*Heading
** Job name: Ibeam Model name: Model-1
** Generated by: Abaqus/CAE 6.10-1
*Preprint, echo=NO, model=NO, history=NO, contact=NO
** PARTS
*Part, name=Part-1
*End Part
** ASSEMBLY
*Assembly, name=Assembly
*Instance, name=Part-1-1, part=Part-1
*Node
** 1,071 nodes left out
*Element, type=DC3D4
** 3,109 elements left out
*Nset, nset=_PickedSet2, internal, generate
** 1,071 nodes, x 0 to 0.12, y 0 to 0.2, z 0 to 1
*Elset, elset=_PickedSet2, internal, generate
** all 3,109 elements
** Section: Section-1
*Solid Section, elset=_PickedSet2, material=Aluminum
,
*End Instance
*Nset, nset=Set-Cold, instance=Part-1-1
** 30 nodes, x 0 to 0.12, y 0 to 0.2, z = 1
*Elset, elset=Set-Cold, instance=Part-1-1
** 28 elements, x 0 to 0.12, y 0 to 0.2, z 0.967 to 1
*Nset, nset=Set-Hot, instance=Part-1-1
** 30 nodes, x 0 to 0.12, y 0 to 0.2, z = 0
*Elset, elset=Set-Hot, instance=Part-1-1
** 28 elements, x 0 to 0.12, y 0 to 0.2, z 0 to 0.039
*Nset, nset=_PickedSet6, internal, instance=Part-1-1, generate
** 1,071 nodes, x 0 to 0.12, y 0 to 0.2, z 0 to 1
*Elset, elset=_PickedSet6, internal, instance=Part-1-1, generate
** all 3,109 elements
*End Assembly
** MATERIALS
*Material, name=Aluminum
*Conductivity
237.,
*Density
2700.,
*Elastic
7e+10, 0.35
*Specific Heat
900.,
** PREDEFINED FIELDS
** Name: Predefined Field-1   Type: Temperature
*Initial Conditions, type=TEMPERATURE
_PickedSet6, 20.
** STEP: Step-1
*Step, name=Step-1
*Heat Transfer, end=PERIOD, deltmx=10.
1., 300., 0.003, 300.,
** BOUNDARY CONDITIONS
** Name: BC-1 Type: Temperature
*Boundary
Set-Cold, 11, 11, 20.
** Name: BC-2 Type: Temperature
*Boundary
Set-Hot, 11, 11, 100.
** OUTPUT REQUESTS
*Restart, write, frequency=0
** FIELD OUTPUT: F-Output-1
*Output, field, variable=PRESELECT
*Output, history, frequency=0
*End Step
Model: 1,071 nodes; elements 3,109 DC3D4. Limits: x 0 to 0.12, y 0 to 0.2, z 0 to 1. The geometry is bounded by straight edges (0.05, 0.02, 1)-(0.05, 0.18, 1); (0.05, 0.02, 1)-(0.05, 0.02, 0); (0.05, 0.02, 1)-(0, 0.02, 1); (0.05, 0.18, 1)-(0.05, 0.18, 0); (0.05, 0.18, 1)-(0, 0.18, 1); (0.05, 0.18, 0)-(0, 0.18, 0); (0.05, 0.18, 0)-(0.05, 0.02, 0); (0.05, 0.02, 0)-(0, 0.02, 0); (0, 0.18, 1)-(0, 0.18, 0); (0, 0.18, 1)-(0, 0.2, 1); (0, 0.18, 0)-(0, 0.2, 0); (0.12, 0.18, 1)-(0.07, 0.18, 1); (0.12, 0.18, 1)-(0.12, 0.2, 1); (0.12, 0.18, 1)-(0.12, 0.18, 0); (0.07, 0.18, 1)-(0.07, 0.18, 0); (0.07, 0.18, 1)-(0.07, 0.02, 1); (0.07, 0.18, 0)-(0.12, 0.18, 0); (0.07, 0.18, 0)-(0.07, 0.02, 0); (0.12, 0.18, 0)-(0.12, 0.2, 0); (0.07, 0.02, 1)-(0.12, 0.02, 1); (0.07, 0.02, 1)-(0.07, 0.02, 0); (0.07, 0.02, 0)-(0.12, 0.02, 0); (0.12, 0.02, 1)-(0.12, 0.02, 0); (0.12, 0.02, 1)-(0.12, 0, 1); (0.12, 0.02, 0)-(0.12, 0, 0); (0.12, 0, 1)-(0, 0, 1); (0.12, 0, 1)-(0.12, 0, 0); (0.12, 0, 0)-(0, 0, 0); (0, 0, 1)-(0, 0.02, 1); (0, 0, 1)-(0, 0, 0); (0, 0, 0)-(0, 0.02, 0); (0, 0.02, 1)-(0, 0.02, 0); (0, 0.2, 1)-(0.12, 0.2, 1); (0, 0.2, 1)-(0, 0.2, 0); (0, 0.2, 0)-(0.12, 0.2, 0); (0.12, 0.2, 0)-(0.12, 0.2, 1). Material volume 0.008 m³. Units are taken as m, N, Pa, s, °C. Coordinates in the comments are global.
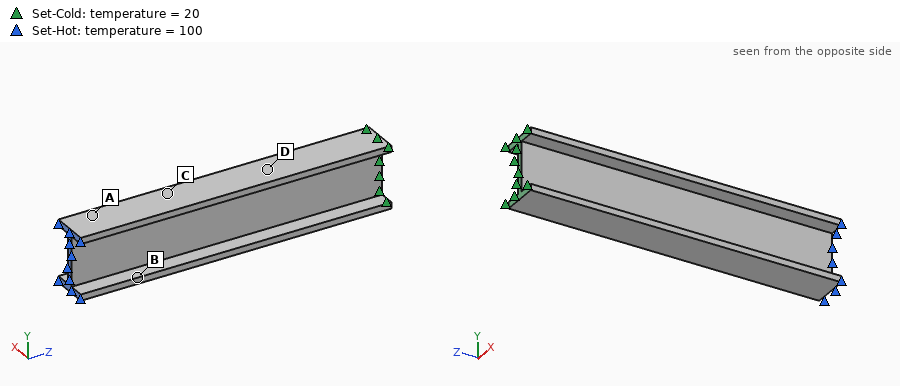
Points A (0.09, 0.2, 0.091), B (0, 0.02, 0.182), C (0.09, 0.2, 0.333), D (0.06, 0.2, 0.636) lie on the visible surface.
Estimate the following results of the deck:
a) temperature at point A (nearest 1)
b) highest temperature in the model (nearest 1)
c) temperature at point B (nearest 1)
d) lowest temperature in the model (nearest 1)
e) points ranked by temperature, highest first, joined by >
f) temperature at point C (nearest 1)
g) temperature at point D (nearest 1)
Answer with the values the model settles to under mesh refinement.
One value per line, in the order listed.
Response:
76 °C
100 °C
56 °C
20 °C
A > B > C > D
33 °C
21 °C
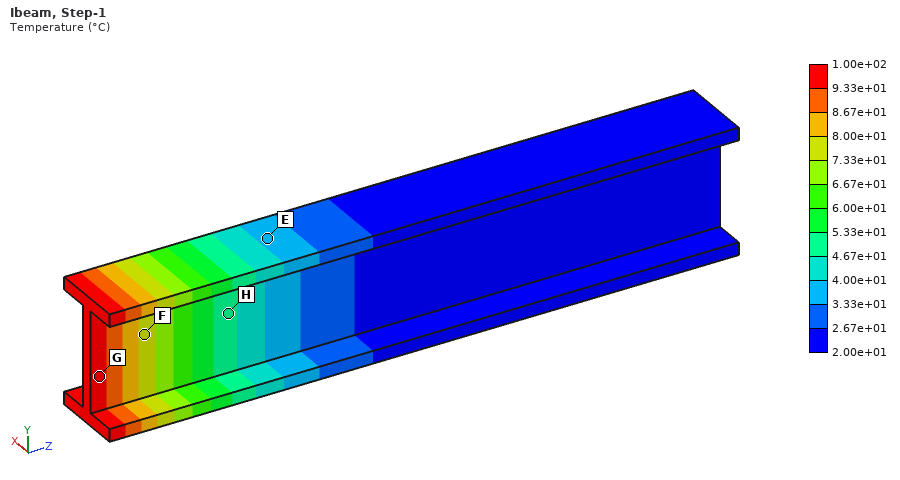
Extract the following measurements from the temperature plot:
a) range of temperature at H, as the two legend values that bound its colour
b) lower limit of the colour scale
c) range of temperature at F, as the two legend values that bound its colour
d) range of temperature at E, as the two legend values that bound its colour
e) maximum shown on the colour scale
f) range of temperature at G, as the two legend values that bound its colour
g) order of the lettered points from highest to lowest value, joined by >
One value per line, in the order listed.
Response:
4.67e+01 to 5.33e+01 °C
2.00e+01 °C
7.33e+01 to 8.00e+01 °C
3.33e+01 to 4.00e+01 °C
1.00e+02 °C
9.33e+01 to 1.00e+02 °C
G > F > H > E
